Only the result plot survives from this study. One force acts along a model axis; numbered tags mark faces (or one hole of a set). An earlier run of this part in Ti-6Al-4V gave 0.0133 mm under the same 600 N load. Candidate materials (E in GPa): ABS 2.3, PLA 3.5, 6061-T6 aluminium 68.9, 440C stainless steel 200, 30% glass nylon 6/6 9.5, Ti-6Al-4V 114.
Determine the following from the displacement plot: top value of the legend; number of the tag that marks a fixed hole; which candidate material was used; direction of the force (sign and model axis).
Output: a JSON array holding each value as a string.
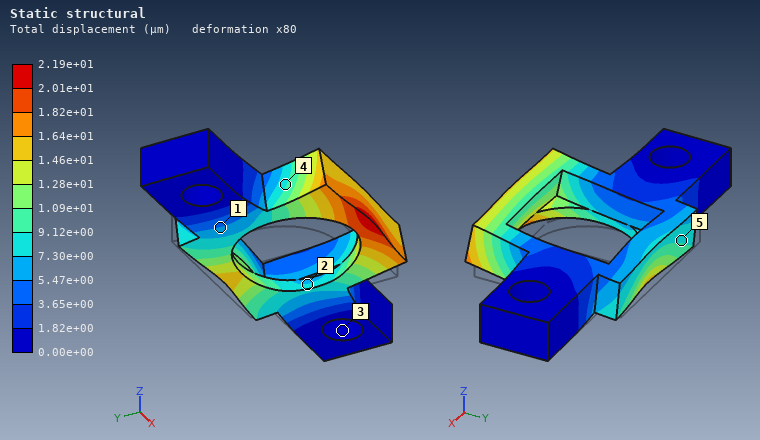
["2.19e+01 µm", "3", "6061-T6 aluminium", "-Y"]
